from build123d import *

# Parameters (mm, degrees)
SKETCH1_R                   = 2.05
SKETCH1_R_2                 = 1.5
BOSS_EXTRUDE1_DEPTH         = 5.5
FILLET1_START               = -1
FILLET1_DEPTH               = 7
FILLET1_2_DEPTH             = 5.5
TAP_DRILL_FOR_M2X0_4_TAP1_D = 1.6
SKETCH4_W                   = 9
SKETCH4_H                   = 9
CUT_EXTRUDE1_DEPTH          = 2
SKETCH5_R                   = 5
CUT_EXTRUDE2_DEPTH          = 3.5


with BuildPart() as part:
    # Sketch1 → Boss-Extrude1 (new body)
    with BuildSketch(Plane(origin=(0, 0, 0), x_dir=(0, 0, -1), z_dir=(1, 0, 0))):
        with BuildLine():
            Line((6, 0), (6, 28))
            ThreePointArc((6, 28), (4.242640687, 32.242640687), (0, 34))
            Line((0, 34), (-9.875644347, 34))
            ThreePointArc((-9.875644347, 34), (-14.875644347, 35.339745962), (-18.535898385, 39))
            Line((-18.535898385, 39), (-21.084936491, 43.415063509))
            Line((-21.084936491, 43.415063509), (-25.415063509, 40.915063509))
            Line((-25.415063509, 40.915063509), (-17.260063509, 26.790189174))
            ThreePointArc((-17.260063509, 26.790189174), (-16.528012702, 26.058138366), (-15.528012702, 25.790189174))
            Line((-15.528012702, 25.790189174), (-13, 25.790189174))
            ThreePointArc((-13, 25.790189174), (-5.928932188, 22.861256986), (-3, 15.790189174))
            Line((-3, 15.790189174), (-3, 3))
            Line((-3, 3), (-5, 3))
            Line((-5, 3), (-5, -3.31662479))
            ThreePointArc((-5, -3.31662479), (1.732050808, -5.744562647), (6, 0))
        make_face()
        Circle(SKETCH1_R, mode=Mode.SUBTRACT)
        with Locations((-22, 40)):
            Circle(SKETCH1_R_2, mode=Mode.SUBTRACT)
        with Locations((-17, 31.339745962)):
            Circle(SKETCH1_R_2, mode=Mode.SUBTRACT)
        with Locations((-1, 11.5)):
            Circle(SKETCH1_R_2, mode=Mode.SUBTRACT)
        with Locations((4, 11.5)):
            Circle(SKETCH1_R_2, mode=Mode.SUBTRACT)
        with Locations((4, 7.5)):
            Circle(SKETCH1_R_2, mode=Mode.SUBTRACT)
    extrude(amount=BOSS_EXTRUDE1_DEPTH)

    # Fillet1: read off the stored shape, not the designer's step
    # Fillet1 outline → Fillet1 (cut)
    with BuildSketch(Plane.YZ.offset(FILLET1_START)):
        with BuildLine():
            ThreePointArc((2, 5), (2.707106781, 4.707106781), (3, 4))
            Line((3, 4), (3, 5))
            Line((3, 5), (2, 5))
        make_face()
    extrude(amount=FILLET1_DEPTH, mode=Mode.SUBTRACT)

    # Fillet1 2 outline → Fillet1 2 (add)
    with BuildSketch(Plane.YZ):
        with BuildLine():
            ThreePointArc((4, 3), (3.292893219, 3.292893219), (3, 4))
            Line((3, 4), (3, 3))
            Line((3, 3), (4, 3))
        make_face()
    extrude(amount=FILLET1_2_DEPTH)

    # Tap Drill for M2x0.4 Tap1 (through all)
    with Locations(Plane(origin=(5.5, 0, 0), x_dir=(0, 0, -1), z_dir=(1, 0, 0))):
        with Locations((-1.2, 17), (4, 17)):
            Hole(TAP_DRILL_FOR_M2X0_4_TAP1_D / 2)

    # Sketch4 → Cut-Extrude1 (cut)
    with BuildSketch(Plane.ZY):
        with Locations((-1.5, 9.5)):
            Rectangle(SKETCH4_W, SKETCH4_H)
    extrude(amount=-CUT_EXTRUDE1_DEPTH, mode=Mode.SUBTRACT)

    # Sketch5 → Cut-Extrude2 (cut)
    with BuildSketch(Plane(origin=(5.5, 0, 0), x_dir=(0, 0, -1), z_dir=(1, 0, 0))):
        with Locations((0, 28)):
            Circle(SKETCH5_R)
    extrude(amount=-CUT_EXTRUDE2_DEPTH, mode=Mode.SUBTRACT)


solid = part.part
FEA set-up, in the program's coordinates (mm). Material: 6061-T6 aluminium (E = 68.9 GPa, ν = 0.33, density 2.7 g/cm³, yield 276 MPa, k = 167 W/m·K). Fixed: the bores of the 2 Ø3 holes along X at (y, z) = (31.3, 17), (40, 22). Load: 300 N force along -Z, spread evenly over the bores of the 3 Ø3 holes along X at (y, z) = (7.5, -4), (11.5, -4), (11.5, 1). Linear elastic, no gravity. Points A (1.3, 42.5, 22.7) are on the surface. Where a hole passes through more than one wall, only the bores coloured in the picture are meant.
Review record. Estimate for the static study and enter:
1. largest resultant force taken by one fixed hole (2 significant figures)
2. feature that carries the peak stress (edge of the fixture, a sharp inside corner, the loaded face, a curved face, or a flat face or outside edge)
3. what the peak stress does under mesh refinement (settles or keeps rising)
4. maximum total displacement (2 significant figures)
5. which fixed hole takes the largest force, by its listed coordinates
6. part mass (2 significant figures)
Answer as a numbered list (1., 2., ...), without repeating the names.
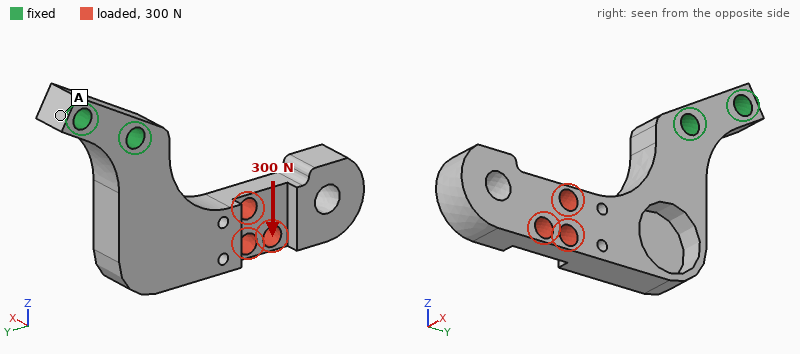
1. 600 N
2. edge of the fixture
3. keeps rising
4. 0.28 mm
5. (31.3, 17)
6. 6.5 g
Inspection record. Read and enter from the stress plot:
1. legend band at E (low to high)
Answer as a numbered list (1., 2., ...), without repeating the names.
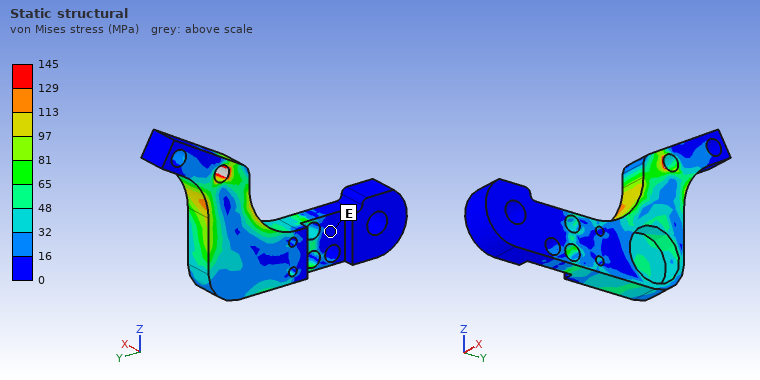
1. 0 to 16 MPa
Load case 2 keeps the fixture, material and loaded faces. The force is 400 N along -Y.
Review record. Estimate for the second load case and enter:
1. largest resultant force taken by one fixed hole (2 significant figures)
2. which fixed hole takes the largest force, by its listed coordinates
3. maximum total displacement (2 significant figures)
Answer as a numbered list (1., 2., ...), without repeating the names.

1. 490 N
2. (31.3, 17)
3. 0.25 mm
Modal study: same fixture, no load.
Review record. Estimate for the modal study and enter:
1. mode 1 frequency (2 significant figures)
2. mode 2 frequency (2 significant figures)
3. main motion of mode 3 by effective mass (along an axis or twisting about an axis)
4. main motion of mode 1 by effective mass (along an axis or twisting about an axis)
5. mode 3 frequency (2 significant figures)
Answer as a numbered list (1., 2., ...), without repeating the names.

1. 1900 Hz
2. 3000 Hz
3. along X
4. along X
5. 6000 Hz
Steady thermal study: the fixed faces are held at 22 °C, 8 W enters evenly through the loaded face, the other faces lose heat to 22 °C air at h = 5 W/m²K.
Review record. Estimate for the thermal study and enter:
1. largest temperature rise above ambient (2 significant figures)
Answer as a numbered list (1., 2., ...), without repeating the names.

1. 43 K
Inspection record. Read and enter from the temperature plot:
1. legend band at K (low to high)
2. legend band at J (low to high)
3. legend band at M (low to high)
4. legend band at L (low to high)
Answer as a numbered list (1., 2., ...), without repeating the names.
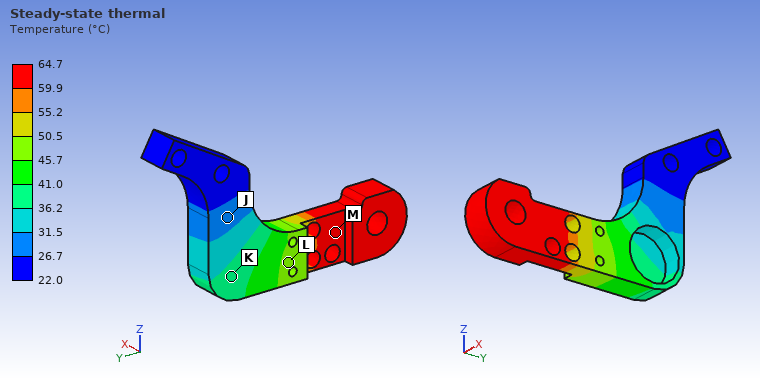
1. 36.2 to 41.0 °C
2. 26.7 to 31.5 °C
3. 59.9 to 64.7 °C
4. 45.7 to 50.5 °C
